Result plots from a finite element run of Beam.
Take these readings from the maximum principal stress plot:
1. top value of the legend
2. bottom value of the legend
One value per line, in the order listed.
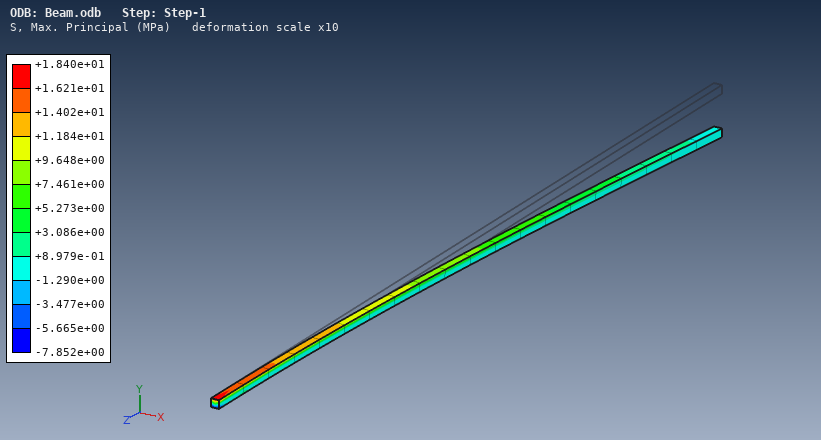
+1.840e+01 MPa
-7.852e+00 MPa
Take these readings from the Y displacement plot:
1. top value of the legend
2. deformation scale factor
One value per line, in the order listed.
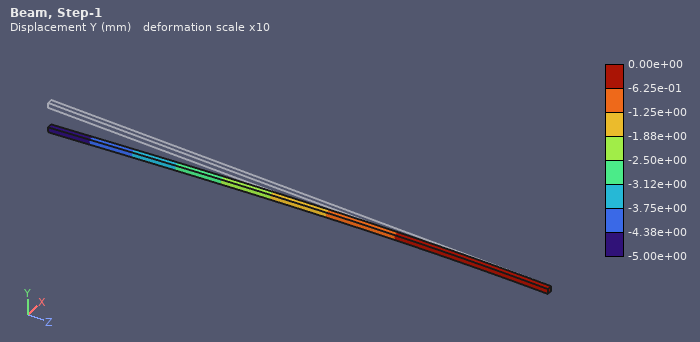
0.00e+00 mm
10
